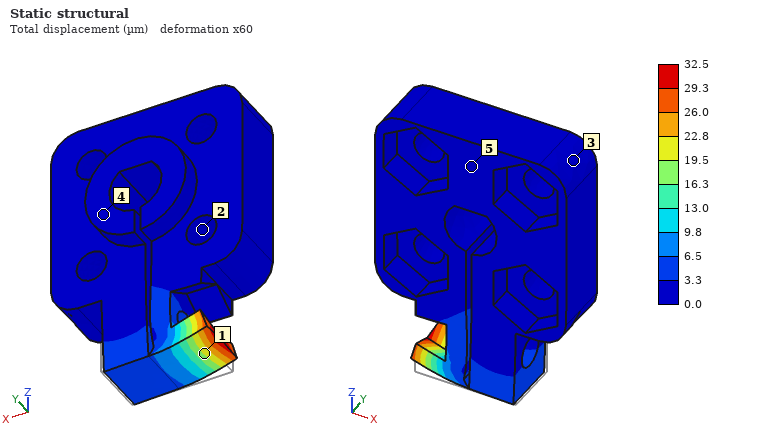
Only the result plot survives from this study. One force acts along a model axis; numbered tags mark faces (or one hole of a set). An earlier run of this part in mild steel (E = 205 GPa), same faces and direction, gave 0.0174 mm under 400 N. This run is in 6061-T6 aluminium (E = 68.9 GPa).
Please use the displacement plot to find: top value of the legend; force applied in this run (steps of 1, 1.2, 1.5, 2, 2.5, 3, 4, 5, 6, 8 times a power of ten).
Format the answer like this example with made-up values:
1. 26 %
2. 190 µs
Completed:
1. 32.5 µm
2. 250 N
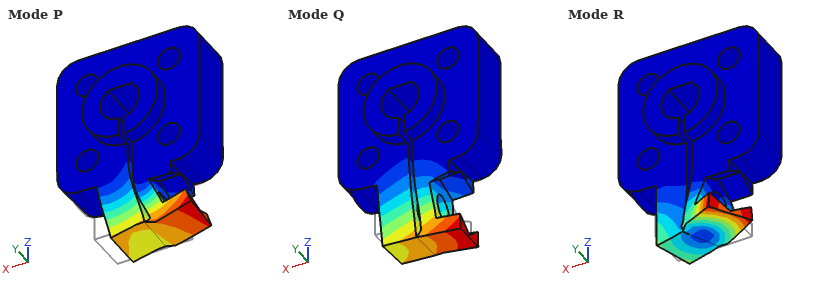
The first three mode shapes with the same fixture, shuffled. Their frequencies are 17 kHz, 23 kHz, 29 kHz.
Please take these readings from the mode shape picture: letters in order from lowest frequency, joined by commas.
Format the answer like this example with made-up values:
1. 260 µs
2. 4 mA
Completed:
1. Q, P, R
